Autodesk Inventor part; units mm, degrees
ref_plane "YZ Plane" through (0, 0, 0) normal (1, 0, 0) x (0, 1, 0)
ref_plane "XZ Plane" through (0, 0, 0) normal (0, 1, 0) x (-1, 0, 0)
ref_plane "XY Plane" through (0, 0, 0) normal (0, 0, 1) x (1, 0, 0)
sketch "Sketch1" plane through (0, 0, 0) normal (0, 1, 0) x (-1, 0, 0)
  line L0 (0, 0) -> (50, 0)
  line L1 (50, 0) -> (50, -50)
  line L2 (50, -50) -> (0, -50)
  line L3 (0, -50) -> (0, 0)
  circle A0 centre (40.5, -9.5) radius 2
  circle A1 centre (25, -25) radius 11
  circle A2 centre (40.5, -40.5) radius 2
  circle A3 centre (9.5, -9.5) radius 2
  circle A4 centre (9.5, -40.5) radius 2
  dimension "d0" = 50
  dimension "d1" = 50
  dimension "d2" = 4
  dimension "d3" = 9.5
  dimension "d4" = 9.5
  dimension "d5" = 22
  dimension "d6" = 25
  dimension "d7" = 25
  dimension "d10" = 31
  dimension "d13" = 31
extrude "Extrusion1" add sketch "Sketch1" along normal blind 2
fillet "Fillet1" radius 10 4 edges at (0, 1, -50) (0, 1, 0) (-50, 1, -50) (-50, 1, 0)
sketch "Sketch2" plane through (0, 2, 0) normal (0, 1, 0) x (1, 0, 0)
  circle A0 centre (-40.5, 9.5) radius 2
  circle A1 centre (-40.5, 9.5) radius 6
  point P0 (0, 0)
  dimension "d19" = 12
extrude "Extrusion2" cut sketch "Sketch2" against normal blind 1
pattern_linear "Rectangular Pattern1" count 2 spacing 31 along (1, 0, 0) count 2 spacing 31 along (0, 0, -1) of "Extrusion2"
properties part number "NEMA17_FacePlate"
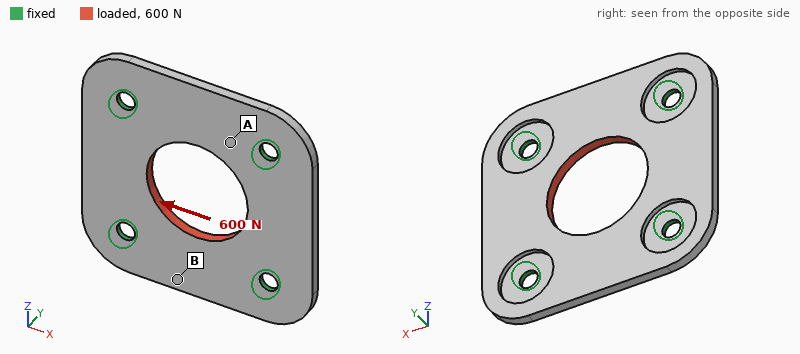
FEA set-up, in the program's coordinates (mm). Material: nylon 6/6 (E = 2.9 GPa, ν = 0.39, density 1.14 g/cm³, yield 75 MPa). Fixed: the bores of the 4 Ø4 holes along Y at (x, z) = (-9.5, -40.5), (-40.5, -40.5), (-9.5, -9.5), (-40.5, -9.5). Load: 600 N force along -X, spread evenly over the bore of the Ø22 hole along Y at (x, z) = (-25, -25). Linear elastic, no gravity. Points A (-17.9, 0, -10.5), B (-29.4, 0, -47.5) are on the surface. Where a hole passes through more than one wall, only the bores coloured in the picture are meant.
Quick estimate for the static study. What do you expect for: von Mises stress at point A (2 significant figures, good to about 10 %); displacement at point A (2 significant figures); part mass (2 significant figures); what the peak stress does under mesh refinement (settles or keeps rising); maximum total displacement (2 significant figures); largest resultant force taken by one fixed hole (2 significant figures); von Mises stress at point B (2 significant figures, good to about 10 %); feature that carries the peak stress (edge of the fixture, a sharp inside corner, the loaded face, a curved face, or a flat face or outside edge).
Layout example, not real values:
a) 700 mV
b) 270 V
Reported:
a) 8.9 MPa
b) 0.028 mm
c) 4.1 g
d) keeps rising
e) 0.11 mm
f) 150 N
g) 1.8 MPa
h) edge of the fixture
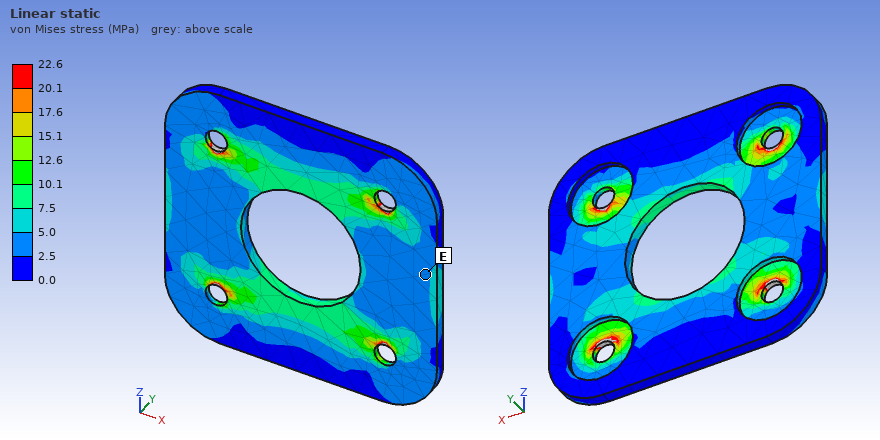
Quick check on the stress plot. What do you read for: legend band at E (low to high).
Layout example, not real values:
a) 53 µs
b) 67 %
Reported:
a) 2.5 to 5.0 MPa
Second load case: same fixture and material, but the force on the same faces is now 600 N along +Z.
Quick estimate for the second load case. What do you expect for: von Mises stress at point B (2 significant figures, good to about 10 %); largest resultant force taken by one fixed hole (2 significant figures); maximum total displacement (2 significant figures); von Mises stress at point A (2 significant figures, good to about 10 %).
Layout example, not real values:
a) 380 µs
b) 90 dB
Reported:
a) 3.9 MPa
b) 150 N
c) 0.11 mm
d) 3.6 MPa
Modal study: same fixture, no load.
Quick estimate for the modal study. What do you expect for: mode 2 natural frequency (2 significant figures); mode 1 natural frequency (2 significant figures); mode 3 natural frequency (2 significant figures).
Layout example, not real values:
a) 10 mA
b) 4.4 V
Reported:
a) 2400 Hz
b) 2100 Hz
c) 2400 Hz
